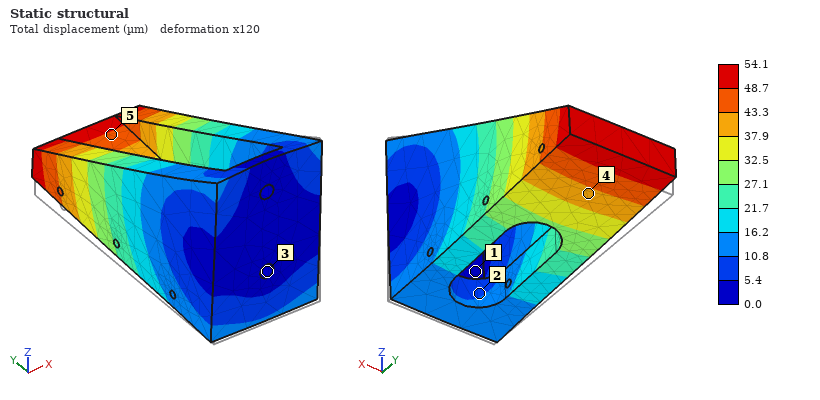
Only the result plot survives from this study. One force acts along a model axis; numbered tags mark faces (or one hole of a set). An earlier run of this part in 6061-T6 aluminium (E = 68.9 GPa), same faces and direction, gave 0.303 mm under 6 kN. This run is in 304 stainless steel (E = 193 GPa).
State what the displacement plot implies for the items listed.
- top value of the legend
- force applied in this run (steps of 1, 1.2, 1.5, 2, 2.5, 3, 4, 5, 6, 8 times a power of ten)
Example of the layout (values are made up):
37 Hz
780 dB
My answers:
54.1 µm
3 kN
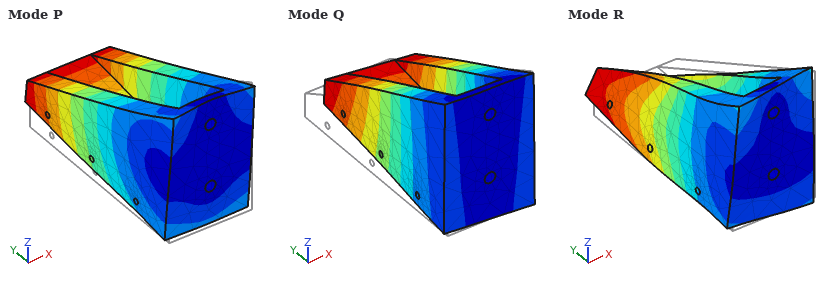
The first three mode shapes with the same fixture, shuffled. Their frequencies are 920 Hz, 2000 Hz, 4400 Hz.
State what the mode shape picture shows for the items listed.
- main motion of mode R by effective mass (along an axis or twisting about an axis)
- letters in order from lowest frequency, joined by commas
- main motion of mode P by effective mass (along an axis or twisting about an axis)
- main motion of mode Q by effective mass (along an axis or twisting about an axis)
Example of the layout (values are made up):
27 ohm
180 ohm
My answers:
twisting about Y
Q, P, R
along Z
along X
